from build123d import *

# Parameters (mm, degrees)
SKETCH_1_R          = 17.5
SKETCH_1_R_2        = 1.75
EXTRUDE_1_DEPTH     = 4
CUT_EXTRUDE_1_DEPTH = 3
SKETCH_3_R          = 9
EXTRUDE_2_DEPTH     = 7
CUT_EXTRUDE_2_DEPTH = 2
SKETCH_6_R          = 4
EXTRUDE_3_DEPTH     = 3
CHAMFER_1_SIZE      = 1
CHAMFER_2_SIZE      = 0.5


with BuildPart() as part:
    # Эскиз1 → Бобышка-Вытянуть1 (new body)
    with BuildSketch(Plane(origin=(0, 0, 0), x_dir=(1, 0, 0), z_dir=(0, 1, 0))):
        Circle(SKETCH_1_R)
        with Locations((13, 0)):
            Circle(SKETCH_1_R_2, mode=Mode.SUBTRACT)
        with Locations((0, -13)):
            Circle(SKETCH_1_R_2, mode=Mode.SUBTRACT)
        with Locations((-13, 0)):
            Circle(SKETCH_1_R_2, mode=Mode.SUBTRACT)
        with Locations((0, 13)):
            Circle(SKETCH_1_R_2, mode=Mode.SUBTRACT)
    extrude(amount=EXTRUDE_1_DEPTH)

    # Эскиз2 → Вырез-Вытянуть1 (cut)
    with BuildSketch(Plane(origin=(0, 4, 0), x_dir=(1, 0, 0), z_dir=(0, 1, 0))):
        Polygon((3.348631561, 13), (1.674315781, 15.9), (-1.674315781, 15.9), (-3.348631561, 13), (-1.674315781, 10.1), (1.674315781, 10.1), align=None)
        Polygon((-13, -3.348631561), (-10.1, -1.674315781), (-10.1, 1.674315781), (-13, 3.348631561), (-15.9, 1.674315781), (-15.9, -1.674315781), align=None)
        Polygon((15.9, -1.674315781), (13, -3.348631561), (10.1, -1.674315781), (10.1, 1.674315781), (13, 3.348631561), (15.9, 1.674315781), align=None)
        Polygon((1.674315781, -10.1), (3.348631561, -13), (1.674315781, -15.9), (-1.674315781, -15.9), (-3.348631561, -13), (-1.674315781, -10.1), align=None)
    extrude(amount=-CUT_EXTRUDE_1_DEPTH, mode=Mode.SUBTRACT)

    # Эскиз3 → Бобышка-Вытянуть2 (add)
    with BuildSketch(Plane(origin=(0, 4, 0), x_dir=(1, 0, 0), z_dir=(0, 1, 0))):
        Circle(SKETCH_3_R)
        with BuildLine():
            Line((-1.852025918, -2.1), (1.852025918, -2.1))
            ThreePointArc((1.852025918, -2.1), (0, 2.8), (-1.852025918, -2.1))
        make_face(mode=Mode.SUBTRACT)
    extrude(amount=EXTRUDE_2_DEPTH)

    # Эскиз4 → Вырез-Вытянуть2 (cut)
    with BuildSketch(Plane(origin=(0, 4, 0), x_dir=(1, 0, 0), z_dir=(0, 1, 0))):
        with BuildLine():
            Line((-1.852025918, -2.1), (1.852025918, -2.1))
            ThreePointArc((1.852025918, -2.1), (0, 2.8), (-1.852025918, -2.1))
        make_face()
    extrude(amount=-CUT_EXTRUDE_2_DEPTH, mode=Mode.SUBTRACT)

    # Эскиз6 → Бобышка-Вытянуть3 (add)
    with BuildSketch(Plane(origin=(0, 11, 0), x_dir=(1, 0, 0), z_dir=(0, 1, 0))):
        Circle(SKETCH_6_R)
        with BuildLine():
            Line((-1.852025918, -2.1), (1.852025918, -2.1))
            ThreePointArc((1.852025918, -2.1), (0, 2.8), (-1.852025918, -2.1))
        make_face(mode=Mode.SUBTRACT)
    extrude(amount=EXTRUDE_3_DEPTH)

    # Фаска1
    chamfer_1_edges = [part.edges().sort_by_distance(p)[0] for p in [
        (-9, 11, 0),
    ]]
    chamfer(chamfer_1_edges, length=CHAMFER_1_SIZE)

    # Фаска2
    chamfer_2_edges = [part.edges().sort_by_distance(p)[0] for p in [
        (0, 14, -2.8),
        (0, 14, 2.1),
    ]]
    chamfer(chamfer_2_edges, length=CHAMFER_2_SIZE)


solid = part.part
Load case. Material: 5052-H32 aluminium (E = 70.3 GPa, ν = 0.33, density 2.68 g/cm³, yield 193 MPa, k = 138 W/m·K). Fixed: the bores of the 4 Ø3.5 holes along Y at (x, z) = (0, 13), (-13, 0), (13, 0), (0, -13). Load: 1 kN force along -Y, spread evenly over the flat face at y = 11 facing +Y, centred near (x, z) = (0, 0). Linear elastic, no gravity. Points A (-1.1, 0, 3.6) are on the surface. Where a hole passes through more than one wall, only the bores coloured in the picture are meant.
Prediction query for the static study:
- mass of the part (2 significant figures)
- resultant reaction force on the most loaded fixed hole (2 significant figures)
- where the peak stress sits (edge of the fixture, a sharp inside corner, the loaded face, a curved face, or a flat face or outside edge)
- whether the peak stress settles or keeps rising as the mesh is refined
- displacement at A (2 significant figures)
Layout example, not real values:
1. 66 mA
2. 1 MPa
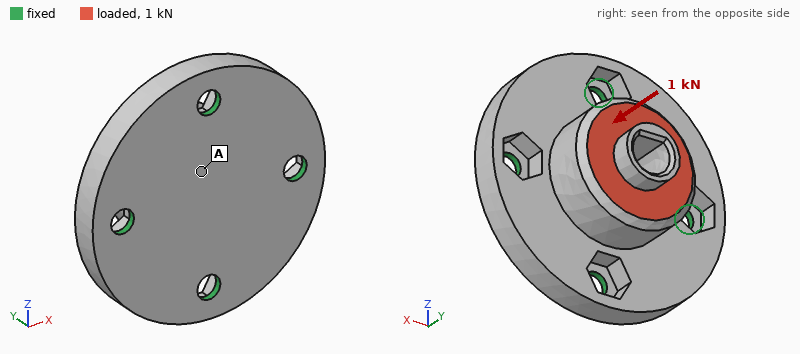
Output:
1. 14 g
2. 290 N
3. edge of the fixture
4. keeps rising
5. 4.9 µm
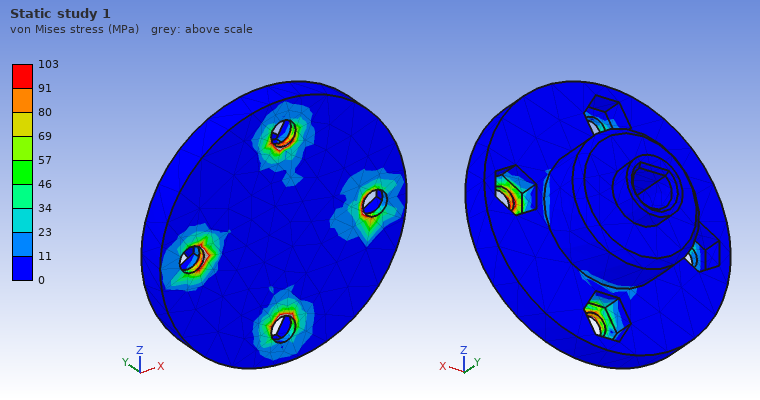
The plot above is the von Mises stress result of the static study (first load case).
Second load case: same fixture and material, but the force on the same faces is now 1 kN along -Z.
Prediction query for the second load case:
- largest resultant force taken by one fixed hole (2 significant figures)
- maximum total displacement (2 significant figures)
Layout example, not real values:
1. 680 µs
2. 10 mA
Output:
1. 560 N
2. 11 µm
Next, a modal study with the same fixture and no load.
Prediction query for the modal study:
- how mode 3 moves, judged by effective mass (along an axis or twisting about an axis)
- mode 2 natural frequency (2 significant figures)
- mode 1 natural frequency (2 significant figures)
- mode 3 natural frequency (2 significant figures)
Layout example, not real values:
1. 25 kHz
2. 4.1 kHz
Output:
1. along Y
2. 22 kHz
3. 22 kHz
4. 23 kHz
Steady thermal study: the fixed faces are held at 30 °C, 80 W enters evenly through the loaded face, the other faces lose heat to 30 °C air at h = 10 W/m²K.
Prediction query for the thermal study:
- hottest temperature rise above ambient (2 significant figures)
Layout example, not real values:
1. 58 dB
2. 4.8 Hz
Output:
1. 54 K
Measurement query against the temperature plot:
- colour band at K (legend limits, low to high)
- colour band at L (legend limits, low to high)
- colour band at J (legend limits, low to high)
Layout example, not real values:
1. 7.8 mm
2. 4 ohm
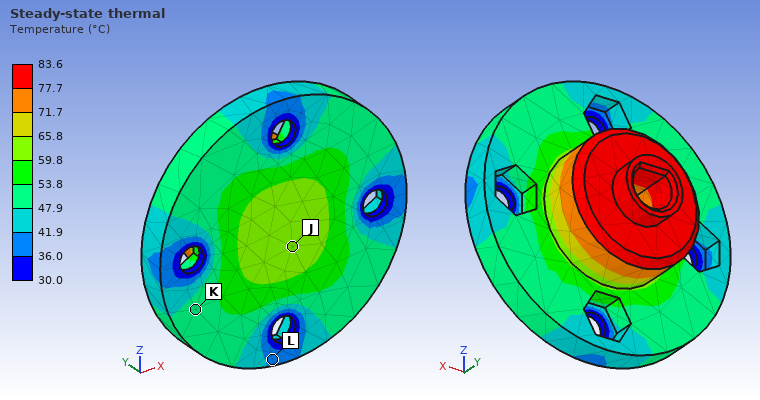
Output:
1. 47.9 to 53.8 °C
2. 36.0 to 41.9 °C
3. 59.8 to 65.8 °C
